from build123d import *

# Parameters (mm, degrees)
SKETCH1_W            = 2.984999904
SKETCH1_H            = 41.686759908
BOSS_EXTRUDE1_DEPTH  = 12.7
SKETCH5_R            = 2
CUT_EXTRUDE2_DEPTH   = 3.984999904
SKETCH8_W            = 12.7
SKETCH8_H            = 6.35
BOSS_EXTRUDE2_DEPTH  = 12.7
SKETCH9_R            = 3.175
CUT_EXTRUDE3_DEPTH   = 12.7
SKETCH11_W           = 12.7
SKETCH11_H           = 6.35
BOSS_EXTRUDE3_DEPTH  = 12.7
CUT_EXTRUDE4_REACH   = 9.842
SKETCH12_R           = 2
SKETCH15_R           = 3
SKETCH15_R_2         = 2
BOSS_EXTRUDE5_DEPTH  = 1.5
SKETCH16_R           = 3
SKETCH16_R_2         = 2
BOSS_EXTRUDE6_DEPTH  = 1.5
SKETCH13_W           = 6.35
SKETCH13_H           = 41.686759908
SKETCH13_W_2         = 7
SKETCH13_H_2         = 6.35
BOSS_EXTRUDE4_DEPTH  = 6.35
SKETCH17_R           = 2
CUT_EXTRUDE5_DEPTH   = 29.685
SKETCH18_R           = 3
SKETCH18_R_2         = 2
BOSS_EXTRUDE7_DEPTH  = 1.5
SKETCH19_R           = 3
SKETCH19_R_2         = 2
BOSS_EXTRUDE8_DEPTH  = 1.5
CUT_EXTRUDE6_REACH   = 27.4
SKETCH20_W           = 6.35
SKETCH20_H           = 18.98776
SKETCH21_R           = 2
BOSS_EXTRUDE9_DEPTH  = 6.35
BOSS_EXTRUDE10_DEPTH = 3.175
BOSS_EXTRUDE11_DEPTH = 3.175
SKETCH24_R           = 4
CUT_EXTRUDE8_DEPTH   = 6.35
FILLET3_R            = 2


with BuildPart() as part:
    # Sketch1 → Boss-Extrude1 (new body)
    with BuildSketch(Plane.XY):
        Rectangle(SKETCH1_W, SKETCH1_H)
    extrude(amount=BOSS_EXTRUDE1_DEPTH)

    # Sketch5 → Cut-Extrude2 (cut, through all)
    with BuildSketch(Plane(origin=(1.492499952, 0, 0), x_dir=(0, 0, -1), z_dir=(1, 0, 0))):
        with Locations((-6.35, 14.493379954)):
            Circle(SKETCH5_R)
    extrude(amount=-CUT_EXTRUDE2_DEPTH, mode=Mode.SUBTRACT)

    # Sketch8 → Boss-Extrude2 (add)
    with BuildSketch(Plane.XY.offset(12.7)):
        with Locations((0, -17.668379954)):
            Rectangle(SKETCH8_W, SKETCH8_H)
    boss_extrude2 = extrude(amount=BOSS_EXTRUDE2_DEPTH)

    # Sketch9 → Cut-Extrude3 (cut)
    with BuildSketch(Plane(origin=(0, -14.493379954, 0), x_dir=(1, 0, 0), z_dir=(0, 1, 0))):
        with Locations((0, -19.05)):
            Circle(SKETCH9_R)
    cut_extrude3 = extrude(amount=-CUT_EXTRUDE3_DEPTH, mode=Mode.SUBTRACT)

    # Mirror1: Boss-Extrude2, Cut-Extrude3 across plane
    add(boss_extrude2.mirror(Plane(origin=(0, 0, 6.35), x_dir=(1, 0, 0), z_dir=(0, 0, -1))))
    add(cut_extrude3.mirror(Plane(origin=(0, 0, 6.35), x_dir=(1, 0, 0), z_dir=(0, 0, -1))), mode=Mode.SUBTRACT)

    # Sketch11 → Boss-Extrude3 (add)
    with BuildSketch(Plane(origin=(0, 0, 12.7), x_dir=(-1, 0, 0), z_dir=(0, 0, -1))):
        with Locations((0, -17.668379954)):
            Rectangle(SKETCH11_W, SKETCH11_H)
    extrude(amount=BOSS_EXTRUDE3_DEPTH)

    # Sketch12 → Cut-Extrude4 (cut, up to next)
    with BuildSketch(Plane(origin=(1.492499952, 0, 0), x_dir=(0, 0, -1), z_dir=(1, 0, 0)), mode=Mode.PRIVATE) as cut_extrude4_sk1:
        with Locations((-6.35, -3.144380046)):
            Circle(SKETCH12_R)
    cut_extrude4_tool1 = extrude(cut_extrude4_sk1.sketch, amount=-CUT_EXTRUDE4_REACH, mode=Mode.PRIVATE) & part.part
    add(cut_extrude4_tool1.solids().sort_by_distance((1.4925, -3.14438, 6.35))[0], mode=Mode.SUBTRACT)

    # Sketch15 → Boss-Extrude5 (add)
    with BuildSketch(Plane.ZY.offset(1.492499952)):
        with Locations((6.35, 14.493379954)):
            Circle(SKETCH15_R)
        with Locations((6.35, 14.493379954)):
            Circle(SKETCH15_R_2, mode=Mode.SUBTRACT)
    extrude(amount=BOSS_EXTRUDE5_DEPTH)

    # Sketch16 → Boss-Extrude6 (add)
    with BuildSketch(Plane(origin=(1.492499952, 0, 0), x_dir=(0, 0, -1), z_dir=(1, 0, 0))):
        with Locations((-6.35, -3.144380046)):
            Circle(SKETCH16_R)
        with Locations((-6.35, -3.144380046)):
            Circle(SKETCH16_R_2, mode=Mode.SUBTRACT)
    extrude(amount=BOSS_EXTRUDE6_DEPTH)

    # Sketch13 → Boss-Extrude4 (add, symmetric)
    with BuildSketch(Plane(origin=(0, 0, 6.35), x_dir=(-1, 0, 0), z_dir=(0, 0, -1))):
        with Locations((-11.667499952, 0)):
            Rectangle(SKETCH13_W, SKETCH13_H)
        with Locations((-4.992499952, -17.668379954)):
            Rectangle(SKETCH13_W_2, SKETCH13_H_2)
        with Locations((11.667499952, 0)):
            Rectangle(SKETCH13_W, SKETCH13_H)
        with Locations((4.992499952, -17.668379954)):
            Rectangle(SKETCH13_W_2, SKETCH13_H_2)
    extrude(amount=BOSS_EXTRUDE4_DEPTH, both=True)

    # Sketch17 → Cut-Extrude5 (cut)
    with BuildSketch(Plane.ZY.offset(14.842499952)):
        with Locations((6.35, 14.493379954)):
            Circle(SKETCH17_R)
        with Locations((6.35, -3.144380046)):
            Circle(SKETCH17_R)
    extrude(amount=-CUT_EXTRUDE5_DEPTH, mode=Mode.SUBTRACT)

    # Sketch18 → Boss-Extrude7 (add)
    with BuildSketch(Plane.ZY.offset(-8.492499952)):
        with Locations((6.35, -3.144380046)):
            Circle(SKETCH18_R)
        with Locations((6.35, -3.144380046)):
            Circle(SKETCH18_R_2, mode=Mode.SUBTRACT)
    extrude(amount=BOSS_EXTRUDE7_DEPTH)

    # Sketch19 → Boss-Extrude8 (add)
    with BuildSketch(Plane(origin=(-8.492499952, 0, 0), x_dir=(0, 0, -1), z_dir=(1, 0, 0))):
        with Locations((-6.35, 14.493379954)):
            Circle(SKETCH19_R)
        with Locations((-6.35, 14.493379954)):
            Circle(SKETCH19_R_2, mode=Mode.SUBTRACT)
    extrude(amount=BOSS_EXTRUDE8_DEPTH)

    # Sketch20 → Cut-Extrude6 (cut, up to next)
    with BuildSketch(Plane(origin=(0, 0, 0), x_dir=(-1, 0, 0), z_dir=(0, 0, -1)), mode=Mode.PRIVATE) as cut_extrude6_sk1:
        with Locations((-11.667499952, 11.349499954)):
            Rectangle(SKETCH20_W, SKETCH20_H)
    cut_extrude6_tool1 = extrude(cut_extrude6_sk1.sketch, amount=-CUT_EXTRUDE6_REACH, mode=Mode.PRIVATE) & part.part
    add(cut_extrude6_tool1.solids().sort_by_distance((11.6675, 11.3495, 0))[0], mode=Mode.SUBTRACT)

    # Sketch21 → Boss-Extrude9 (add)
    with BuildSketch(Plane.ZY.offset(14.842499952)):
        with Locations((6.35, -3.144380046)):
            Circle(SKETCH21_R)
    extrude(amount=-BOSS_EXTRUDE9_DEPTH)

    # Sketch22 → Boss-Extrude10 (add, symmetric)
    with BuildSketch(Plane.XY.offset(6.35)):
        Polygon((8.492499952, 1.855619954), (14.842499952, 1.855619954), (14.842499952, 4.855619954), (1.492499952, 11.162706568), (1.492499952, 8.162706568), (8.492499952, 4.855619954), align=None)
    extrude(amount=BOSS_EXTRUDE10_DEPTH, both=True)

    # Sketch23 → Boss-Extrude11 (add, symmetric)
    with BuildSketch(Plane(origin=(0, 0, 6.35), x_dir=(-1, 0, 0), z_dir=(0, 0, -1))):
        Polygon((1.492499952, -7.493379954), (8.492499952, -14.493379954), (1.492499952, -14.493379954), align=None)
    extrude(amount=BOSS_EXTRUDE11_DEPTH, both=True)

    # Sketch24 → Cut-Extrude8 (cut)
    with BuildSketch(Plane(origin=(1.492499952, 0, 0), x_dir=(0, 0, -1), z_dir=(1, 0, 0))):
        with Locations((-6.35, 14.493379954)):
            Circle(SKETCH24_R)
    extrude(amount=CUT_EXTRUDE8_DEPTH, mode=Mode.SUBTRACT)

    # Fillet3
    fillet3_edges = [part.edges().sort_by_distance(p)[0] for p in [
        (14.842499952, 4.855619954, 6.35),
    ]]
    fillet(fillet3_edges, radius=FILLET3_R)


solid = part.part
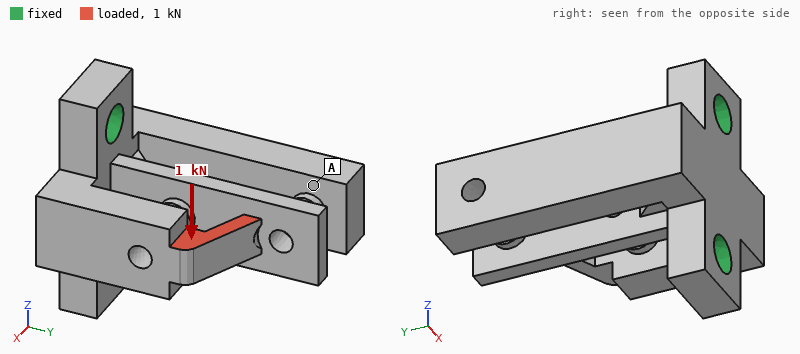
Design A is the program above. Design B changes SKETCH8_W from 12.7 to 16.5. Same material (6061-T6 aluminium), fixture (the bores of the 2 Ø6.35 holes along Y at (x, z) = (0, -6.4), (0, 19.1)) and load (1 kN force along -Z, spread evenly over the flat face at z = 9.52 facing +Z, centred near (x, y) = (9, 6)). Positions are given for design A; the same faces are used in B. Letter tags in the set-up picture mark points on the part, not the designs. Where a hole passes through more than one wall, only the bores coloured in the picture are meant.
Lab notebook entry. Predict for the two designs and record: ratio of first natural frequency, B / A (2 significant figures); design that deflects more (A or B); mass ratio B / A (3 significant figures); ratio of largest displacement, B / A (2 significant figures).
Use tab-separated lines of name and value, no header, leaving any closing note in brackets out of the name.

ratio of first natural frequency, B / A	1.0
design that deflects more	A
mass ratio B / A	1.06
ratio of largest displacement, B / A	0.91
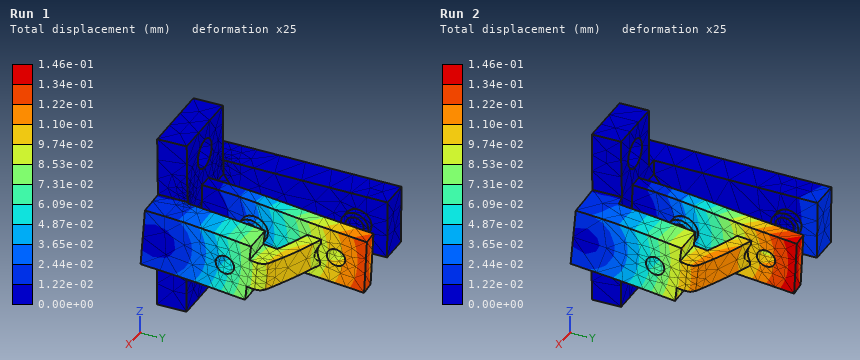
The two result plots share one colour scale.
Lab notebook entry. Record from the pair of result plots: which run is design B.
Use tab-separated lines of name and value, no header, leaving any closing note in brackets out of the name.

which run is design B	Run 1
